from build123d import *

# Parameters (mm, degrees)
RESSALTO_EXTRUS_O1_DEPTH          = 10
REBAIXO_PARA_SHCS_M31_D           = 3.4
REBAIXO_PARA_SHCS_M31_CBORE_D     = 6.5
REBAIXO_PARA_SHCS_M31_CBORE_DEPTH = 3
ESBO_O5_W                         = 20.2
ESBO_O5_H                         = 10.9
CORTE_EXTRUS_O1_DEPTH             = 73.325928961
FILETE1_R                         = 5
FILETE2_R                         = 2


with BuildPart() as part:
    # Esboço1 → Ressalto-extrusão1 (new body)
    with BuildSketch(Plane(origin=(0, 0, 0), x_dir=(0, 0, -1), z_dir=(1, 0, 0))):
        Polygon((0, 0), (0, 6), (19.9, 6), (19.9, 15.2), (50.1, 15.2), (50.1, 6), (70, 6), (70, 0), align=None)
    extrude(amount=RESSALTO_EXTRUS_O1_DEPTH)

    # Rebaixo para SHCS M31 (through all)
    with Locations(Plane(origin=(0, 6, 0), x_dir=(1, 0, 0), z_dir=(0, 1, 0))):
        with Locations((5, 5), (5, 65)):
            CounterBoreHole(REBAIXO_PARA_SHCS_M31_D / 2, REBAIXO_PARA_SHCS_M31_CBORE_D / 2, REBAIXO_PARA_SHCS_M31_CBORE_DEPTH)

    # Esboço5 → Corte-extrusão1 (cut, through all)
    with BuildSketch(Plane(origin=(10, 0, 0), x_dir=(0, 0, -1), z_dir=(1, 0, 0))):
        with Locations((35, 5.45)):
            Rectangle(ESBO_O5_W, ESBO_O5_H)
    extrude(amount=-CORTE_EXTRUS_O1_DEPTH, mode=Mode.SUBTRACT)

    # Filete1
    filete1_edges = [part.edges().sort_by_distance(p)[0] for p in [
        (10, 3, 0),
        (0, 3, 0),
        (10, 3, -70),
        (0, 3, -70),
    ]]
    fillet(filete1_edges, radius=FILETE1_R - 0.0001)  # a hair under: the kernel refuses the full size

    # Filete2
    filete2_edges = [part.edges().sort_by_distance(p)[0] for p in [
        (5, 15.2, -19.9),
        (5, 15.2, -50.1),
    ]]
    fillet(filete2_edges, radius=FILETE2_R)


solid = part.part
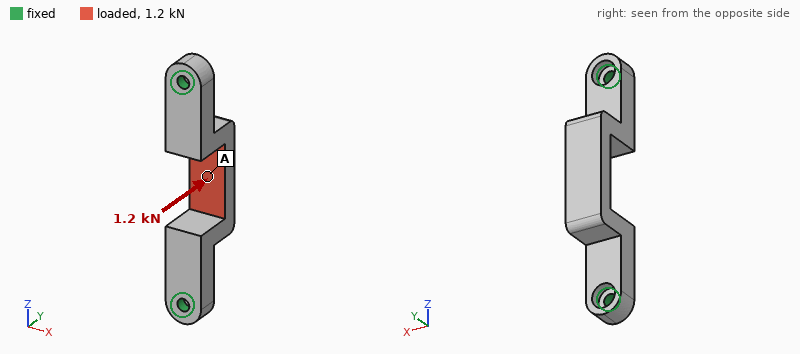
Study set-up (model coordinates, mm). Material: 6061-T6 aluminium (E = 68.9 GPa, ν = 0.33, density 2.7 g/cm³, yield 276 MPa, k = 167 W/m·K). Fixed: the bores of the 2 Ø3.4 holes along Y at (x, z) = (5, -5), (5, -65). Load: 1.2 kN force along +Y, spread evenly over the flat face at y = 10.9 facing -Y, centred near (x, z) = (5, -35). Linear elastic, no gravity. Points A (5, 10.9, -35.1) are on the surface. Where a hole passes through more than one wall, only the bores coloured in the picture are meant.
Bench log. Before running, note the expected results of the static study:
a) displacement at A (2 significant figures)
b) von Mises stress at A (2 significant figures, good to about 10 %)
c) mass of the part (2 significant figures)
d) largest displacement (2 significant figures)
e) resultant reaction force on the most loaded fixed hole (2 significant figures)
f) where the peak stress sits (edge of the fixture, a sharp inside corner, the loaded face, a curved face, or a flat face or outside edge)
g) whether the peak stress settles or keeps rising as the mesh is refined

62 µm
19 MPa
12 g
63 µm
1.1 kN
edge of the fixture
keeps rising
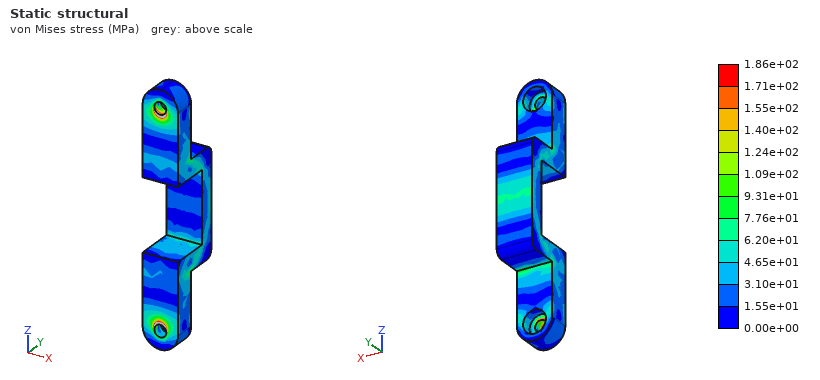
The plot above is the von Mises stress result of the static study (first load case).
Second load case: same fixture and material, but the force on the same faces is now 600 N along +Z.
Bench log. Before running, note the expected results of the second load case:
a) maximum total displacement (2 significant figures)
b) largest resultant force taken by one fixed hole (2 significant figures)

17 µm
310 N
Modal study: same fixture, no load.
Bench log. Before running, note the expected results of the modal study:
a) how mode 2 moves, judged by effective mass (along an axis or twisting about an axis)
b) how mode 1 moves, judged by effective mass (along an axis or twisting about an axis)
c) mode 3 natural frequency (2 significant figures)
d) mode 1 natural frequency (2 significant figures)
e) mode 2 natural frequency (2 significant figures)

along Y
along X
10 kHz
5500 Hz
8700 Hz
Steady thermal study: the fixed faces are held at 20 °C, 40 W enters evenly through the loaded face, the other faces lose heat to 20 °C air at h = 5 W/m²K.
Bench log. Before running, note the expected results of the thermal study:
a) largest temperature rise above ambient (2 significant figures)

74 K
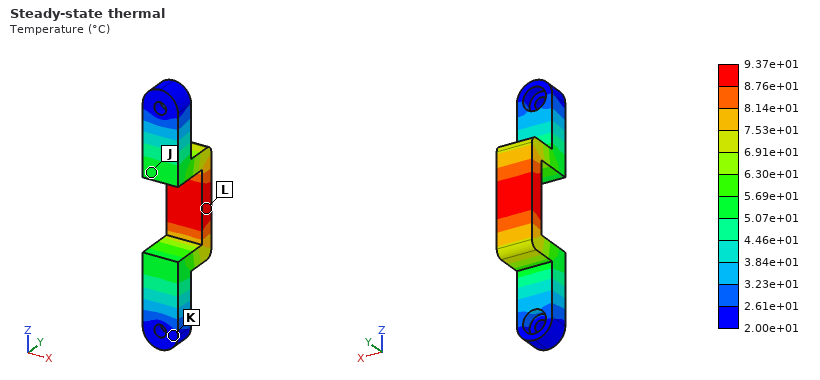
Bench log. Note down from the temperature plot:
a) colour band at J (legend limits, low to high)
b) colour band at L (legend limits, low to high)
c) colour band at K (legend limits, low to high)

5.07e+01 to 5.69e+01 °C
8.76e+01 to 9.37e+01 °C
2.00e+01 to 2.61e+01 °C
